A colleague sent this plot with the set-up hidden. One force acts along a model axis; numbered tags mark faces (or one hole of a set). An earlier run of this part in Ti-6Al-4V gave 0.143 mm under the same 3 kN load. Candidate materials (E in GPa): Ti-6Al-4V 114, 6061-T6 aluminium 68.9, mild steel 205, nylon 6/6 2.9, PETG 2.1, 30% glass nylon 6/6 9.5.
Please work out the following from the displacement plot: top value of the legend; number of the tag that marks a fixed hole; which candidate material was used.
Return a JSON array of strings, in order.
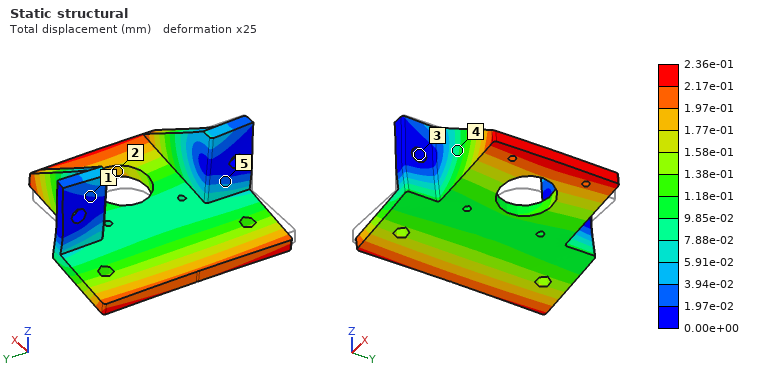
["2.36e-01 mm", "3", "6061-T6 aluminium"]
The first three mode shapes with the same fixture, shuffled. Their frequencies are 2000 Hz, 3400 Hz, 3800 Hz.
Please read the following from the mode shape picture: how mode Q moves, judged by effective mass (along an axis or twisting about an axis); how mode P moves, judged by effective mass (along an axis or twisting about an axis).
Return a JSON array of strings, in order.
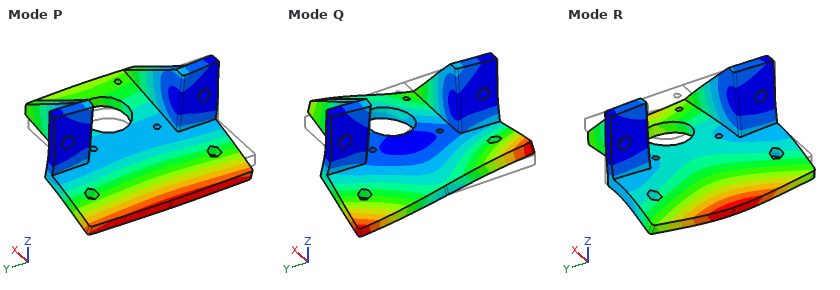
["twisting about Z", "along X"]
